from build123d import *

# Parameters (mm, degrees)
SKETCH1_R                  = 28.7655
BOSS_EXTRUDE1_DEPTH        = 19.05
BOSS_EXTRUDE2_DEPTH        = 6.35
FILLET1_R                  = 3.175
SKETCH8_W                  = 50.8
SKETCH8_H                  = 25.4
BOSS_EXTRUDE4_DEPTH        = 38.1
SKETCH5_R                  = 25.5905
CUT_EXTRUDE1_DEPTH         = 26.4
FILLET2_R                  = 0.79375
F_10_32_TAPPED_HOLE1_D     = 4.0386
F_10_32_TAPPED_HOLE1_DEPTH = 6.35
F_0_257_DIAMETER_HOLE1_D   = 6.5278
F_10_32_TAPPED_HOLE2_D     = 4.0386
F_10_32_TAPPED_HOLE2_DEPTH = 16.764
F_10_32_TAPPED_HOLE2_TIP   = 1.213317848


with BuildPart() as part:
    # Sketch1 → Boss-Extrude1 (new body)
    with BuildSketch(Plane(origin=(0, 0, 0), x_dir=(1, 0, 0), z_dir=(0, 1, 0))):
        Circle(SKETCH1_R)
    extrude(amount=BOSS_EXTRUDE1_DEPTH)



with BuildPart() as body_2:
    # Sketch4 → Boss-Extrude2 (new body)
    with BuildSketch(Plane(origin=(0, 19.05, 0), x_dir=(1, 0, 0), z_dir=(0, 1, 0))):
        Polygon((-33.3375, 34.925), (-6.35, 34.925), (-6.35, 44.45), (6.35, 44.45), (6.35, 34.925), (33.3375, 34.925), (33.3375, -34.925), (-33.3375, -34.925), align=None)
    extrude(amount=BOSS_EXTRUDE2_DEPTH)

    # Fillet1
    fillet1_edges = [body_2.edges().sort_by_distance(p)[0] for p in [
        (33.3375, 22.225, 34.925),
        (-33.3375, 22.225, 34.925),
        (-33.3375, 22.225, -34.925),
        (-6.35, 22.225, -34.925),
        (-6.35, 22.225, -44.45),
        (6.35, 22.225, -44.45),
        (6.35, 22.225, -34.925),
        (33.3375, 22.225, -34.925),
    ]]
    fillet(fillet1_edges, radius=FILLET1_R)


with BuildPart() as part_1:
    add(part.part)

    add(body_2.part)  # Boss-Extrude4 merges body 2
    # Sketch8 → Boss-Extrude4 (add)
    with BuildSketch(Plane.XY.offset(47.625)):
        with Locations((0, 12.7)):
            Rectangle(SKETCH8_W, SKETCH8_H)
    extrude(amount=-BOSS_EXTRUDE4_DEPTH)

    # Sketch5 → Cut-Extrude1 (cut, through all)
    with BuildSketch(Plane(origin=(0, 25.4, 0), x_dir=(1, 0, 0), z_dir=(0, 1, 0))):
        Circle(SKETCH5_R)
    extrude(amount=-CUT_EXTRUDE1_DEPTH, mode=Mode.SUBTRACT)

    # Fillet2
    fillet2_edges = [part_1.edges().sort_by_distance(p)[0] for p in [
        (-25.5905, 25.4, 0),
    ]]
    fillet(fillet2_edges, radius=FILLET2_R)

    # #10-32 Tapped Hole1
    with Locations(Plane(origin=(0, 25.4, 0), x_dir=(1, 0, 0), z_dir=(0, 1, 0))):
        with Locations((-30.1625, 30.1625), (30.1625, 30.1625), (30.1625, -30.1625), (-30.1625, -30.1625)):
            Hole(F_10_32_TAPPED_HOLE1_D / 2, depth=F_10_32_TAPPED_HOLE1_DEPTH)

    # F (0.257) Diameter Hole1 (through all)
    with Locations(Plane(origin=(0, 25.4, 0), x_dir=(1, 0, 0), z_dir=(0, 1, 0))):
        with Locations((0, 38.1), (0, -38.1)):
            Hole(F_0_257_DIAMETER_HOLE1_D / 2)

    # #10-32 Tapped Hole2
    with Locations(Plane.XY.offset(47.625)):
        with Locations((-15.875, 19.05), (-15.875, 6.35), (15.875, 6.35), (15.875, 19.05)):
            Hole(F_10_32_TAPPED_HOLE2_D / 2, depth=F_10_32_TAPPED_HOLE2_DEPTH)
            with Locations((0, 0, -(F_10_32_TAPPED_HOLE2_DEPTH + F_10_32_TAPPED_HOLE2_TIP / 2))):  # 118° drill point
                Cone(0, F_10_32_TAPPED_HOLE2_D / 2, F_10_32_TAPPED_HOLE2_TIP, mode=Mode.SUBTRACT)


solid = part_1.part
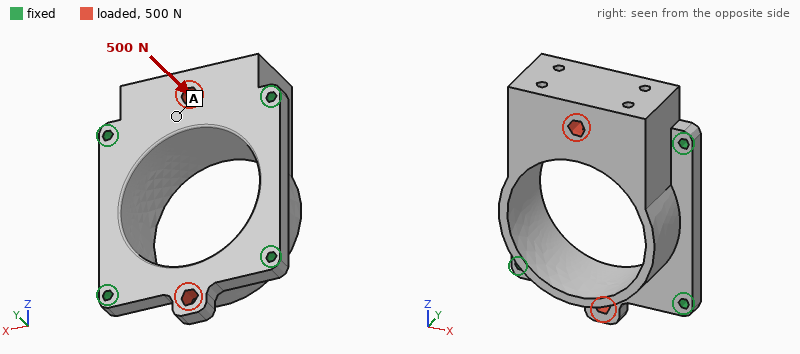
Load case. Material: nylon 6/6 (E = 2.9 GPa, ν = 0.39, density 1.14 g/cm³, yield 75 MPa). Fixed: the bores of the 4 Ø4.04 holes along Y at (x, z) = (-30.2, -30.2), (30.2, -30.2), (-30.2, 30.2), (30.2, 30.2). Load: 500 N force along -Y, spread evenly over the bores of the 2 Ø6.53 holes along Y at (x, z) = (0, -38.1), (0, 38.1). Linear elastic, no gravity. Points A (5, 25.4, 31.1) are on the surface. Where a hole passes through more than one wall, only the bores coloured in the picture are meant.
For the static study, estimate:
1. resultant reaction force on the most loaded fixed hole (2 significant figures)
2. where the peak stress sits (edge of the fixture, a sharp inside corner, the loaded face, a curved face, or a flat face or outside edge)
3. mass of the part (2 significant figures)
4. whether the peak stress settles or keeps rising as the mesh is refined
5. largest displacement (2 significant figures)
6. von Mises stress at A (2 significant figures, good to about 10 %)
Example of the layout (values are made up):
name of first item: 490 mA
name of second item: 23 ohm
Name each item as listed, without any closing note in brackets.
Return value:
resultant reaction force on the most loaded fixed hole: 260 N
where the peak stress sits: edge of the fixture
mass of the part: 59 g
whether the peak stress settles or keeps rising as the mesh is refined: keeps rising
largest displacement: 0.30 mm
von Mises stress at A: 1.4 MPa
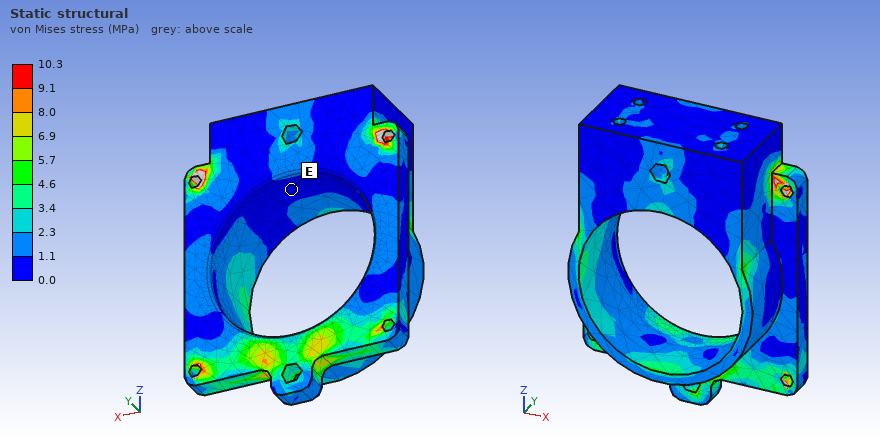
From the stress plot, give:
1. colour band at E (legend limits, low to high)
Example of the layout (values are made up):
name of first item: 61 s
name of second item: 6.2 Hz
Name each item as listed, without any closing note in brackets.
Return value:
colour band at E: 0.0 to 1.1 MPa
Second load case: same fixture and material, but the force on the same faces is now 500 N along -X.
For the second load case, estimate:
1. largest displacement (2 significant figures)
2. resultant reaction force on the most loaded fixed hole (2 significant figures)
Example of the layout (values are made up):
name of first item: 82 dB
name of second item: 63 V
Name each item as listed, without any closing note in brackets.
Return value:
largest displacement: 34 µm
resultant reaction force on the most loaded fixed hole: 220 N
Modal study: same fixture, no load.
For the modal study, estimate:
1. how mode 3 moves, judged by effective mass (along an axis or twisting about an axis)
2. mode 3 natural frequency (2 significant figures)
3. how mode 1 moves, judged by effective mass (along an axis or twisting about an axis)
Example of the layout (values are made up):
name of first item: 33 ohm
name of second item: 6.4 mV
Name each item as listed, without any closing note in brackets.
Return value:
how mode 3 moves, judged by effective mass: along Y
mode 3 natural frequency: 2700 Hz
how mode 1 moves, judged by effective mass: along Z
